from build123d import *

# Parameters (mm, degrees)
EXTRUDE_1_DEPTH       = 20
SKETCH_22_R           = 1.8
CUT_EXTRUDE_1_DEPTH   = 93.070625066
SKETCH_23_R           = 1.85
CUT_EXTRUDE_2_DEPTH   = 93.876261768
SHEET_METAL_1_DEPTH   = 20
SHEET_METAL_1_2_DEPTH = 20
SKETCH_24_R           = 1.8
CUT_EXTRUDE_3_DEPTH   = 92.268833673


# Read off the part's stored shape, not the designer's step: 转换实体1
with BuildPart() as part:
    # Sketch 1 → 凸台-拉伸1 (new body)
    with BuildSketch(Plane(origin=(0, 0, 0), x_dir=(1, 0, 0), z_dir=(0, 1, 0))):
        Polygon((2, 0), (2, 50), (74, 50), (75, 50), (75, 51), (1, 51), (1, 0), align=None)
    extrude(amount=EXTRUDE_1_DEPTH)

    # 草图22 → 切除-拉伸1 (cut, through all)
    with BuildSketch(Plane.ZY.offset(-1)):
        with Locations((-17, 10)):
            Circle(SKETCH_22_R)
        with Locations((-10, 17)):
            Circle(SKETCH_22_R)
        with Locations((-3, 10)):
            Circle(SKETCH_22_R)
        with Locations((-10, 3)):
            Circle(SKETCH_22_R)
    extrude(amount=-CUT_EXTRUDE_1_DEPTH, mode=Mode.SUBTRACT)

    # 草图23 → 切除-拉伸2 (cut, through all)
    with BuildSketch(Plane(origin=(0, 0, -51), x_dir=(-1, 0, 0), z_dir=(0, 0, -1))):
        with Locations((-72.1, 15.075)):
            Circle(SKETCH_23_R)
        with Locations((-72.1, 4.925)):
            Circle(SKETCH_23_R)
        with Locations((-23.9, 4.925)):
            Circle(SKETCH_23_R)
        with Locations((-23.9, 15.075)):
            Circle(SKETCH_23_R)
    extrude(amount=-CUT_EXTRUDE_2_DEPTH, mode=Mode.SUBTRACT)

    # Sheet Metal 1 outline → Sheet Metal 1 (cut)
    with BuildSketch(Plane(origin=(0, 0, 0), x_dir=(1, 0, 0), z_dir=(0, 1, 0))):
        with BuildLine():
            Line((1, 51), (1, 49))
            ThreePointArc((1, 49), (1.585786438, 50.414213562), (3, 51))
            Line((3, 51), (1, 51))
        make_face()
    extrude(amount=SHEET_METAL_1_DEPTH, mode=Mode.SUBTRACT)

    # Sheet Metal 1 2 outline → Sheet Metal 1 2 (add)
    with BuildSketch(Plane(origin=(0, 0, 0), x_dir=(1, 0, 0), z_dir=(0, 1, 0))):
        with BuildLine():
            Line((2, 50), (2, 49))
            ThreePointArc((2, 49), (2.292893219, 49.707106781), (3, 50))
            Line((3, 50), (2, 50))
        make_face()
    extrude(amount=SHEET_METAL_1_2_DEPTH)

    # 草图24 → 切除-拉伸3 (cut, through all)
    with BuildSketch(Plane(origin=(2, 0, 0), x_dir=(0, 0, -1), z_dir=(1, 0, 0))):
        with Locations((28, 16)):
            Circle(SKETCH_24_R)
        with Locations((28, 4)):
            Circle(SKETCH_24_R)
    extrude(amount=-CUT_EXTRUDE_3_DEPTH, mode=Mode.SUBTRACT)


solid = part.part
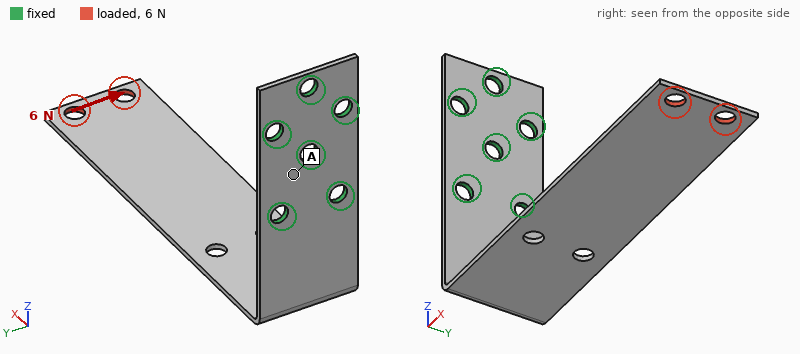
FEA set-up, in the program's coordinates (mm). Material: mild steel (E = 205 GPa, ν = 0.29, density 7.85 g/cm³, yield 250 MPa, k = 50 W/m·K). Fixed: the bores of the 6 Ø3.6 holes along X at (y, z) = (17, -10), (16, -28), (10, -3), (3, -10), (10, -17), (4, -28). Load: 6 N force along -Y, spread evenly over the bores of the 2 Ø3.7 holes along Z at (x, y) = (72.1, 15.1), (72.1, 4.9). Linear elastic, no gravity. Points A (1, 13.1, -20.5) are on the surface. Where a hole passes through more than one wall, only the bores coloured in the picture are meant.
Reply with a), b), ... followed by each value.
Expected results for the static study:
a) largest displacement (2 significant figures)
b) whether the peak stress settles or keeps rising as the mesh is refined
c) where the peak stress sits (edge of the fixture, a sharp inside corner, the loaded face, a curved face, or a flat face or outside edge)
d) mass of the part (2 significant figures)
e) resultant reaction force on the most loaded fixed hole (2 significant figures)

a) 0.88 mm
b) keeps rising
c) edge of the fixture
d) 19 g
e) 31 N
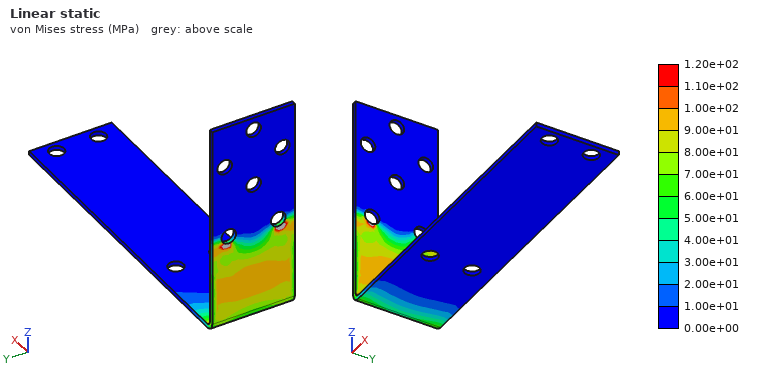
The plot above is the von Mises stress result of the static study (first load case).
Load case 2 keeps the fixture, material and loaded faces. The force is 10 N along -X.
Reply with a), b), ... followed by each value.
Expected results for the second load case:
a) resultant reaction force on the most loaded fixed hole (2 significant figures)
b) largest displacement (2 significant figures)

a) 5.5 N
b) 0.48 mm
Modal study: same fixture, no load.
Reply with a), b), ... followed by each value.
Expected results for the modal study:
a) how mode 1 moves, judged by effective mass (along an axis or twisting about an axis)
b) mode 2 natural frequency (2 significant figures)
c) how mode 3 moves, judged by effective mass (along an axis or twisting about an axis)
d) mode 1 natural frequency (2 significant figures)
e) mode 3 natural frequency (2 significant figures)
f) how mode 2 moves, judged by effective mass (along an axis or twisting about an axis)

a) along Z
b) 210 Hz
c) along X
d) 110 Hz
e) 560 Hz
f) along Y
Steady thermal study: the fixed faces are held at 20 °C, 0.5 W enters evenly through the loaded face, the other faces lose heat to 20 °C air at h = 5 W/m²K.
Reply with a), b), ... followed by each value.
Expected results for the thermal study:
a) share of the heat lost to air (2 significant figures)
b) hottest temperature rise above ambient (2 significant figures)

a) 53 %
b) 31 K
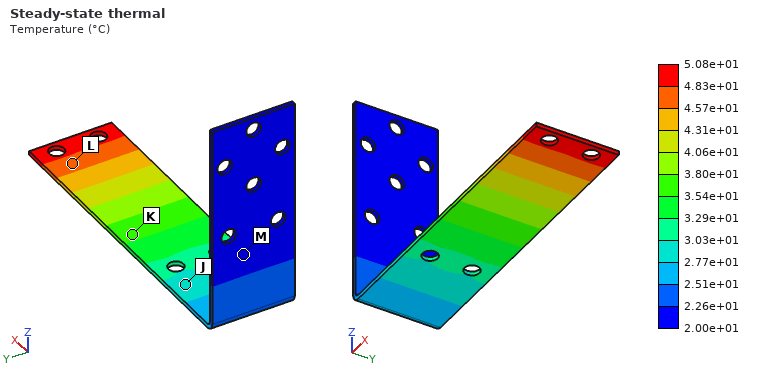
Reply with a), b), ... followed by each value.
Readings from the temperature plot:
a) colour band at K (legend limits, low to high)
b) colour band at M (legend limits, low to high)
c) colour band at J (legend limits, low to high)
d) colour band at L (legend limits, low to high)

a) 3.54e+01 to 3.80e+01 °C
b) 2.00e+01 to 2.26e+01 °C
c) 2.77e+01 to 3.03e+01 °C
d) 4.57e+01 to 4.83e+01 °C
